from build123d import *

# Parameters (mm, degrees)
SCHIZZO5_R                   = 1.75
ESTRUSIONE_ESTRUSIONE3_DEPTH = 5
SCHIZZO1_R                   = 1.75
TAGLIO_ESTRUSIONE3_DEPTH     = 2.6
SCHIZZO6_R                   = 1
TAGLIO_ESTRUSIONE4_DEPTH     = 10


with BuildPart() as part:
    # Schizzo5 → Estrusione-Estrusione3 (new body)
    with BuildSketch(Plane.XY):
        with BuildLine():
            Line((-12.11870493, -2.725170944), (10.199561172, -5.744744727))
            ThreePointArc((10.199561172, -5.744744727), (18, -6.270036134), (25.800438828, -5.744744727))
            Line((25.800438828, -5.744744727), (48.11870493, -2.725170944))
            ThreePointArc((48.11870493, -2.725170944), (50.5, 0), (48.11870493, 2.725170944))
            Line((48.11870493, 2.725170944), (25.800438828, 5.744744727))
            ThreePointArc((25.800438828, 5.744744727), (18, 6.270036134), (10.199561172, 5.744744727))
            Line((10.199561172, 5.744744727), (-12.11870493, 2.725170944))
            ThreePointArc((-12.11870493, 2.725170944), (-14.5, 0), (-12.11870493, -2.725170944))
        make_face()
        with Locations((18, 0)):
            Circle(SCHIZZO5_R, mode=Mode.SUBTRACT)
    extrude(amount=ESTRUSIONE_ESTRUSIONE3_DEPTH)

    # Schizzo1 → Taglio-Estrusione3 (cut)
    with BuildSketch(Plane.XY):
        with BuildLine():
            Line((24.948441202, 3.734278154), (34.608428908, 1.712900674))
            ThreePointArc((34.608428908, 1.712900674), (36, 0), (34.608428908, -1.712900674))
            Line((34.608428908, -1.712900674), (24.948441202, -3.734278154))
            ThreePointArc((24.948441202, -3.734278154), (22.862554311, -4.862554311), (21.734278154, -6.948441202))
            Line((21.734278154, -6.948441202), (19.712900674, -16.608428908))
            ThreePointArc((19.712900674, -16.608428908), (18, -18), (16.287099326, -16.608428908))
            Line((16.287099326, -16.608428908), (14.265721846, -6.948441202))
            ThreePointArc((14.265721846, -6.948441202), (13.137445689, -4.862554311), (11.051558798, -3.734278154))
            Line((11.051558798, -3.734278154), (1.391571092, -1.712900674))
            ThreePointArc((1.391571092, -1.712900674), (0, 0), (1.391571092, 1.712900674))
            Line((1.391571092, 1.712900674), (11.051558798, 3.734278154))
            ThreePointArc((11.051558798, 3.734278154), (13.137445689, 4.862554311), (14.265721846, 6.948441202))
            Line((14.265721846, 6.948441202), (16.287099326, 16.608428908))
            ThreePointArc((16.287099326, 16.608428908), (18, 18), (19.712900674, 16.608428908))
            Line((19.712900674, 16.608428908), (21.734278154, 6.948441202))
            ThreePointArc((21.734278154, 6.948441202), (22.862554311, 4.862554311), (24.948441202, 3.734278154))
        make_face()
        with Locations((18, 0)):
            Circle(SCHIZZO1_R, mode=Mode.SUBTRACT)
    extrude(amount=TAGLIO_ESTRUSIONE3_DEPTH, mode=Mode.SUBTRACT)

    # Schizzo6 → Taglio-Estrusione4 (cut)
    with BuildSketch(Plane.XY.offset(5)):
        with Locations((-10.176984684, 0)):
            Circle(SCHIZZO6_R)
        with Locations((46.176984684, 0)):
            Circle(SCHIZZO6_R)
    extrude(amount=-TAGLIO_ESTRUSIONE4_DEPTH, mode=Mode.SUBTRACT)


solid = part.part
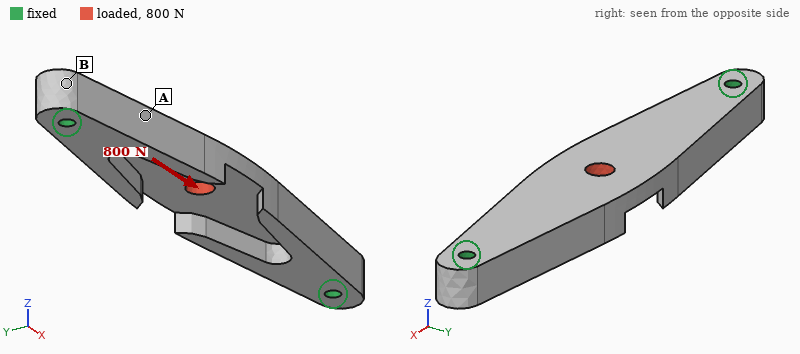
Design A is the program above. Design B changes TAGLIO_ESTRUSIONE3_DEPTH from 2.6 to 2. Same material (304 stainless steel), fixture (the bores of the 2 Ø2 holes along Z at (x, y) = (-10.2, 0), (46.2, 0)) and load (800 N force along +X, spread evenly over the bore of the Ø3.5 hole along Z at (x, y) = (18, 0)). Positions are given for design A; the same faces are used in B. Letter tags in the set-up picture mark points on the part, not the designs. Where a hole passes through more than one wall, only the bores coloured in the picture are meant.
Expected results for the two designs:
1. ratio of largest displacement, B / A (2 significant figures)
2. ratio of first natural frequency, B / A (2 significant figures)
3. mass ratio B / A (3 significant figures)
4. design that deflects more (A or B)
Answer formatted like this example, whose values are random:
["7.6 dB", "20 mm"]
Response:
["0.86", "0.97", "1.07", "A"]
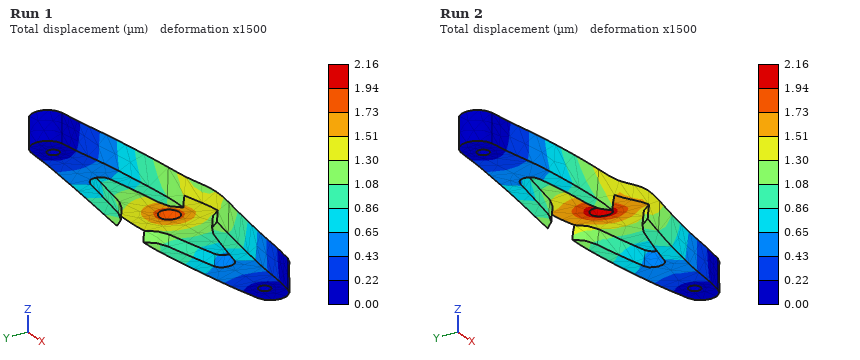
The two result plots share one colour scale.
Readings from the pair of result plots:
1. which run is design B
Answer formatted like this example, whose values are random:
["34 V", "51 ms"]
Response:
["Run 1"]
